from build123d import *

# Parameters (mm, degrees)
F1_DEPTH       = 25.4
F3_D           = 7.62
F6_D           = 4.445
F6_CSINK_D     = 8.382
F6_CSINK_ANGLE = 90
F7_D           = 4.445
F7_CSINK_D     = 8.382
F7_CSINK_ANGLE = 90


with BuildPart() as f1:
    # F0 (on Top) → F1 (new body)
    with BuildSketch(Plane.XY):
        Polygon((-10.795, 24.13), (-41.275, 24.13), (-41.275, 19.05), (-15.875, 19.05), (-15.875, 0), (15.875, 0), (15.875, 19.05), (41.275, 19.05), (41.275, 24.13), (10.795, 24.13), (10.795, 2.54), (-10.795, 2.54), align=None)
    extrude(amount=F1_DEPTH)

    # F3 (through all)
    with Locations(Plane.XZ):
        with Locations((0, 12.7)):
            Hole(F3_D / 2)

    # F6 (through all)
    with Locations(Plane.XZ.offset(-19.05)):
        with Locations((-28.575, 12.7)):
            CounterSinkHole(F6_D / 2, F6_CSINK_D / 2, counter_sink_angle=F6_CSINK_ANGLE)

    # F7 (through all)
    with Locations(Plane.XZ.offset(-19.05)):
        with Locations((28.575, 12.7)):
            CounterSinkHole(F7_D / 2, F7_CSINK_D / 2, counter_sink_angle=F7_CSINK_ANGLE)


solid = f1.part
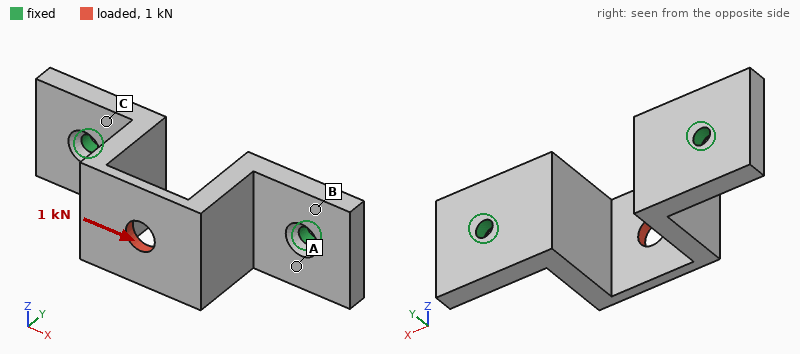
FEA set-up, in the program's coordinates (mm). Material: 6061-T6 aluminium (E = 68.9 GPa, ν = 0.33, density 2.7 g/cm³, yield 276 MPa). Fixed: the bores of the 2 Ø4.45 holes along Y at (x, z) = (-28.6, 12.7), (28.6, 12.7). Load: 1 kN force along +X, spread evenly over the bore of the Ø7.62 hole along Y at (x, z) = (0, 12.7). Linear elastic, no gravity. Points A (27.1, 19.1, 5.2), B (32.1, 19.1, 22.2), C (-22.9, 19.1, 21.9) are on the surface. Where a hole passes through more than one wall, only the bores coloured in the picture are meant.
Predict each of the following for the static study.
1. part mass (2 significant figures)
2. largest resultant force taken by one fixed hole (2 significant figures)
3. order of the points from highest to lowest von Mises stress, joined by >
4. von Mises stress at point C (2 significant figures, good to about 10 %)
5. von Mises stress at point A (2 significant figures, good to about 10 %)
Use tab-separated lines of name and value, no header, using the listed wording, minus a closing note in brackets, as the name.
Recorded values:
part mass	37 g
largest resultant force taken by one fixed hole	590 N
order of the points from highest to lowest von Mises stress, joined by >	C > A > B
von Mises stress at point C	29 MPa
von Mises stress at point A	17 MPa
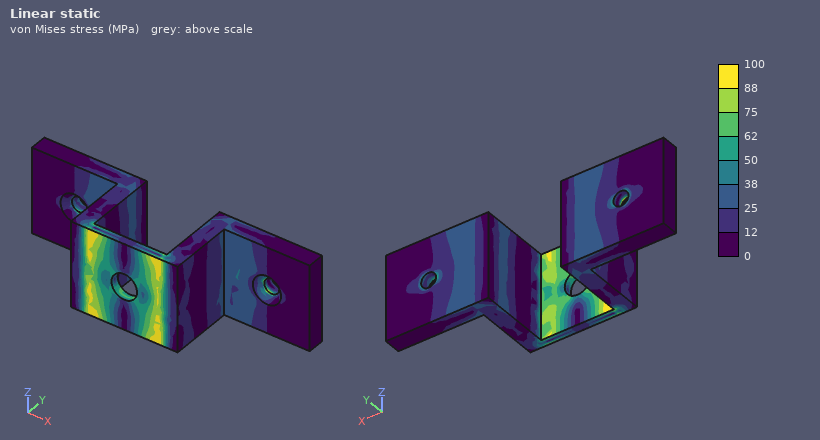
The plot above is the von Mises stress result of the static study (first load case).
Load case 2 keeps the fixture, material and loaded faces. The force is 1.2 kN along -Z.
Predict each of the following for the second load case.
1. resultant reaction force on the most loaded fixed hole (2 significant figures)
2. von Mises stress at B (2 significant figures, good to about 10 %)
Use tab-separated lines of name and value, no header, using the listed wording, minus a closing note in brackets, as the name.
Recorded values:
resultant reaction force on the most loaded fixed hole	600 N
von Mises stress at B	45 MPa
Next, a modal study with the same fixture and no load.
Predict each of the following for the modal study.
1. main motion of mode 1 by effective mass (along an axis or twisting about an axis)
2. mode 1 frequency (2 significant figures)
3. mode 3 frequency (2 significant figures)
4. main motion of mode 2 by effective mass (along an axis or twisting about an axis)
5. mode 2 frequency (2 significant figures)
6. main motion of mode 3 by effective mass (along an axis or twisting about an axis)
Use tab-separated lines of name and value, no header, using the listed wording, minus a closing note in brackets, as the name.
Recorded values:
main motion of mode 1 by effective mass	along Z
mode 1 frequency	3500 Hz
mode 3 frequency	6800 Hz
main motion of mode 2 by effective mass	along X
mode 2 frequency	4900 Hz
main motion of mode 3 by effective mass	along Y
